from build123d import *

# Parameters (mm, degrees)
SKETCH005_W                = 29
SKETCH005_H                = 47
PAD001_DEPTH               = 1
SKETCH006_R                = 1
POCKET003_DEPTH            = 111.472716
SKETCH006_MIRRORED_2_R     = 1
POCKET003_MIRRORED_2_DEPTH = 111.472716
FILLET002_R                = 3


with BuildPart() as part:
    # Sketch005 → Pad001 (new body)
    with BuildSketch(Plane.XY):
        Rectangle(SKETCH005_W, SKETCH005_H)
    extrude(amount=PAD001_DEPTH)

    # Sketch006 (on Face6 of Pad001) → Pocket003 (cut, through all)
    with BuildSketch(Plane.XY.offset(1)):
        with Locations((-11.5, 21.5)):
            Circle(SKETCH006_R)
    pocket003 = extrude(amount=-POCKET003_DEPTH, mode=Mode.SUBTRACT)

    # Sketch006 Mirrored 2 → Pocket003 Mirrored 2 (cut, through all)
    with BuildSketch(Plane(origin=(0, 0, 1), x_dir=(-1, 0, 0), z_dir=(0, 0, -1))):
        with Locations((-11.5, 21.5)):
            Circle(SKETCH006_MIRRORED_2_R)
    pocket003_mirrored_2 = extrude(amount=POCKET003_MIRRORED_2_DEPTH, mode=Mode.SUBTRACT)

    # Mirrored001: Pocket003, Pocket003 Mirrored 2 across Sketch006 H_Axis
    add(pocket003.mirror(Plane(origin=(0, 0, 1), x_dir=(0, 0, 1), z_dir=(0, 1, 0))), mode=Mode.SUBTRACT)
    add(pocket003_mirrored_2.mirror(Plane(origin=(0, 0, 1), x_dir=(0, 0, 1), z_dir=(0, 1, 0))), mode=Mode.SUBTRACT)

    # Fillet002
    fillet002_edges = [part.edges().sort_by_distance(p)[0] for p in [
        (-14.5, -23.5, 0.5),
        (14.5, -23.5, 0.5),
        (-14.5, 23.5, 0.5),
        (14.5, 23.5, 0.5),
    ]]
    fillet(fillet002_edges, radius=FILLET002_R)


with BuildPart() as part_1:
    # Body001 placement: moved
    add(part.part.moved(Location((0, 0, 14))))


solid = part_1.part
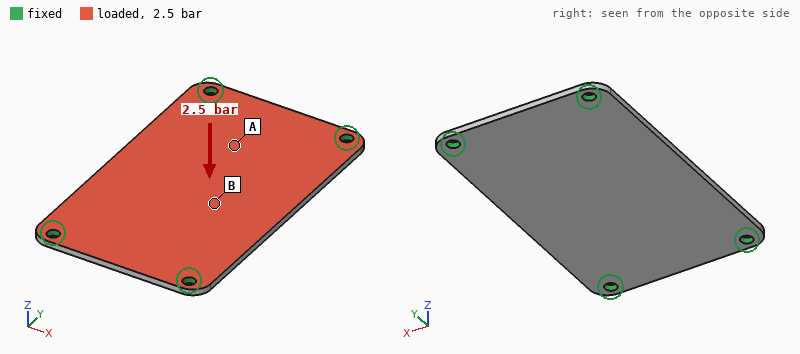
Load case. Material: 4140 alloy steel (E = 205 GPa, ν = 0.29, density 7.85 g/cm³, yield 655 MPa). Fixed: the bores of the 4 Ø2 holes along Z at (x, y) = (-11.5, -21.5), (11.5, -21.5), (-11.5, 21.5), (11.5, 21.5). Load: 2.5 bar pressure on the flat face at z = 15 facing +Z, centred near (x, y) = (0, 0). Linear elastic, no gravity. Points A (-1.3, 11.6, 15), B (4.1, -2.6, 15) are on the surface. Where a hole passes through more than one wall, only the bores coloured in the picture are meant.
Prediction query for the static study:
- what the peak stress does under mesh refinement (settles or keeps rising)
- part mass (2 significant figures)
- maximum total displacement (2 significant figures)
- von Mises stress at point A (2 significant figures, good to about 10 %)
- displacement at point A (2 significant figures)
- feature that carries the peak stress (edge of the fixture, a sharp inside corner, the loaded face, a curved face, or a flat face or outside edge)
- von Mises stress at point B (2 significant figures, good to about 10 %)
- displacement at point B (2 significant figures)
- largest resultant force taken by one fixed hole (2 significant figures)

keeps rising
11 g
0.16 mm
46 MPa
0.098 mm
edge of the fixture
110 MPa
0.16 mm
84 N
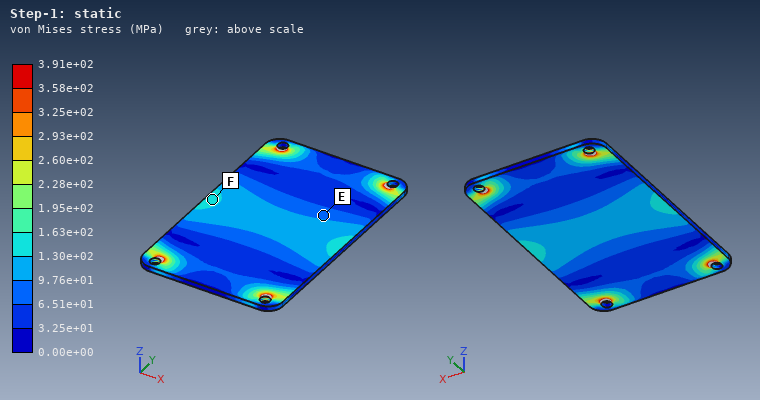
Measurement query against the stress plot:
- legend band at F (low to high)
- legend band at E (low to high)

1.30e+02 to 1.63e+02 MPa
6.51e+01 to 9.76e+01 MPa
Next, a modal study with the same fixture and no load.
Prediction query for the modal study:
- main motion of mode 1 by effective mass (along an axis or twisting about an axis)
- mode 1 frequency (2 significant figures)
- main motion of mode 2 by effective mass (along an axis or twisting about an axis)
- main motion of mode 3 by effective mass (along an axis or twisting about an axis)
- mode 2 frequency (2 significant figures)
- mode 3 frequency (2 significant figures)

along Z
2600 Hz
twisting about Y
twisting about X
4100 Hz
6800 Hz
